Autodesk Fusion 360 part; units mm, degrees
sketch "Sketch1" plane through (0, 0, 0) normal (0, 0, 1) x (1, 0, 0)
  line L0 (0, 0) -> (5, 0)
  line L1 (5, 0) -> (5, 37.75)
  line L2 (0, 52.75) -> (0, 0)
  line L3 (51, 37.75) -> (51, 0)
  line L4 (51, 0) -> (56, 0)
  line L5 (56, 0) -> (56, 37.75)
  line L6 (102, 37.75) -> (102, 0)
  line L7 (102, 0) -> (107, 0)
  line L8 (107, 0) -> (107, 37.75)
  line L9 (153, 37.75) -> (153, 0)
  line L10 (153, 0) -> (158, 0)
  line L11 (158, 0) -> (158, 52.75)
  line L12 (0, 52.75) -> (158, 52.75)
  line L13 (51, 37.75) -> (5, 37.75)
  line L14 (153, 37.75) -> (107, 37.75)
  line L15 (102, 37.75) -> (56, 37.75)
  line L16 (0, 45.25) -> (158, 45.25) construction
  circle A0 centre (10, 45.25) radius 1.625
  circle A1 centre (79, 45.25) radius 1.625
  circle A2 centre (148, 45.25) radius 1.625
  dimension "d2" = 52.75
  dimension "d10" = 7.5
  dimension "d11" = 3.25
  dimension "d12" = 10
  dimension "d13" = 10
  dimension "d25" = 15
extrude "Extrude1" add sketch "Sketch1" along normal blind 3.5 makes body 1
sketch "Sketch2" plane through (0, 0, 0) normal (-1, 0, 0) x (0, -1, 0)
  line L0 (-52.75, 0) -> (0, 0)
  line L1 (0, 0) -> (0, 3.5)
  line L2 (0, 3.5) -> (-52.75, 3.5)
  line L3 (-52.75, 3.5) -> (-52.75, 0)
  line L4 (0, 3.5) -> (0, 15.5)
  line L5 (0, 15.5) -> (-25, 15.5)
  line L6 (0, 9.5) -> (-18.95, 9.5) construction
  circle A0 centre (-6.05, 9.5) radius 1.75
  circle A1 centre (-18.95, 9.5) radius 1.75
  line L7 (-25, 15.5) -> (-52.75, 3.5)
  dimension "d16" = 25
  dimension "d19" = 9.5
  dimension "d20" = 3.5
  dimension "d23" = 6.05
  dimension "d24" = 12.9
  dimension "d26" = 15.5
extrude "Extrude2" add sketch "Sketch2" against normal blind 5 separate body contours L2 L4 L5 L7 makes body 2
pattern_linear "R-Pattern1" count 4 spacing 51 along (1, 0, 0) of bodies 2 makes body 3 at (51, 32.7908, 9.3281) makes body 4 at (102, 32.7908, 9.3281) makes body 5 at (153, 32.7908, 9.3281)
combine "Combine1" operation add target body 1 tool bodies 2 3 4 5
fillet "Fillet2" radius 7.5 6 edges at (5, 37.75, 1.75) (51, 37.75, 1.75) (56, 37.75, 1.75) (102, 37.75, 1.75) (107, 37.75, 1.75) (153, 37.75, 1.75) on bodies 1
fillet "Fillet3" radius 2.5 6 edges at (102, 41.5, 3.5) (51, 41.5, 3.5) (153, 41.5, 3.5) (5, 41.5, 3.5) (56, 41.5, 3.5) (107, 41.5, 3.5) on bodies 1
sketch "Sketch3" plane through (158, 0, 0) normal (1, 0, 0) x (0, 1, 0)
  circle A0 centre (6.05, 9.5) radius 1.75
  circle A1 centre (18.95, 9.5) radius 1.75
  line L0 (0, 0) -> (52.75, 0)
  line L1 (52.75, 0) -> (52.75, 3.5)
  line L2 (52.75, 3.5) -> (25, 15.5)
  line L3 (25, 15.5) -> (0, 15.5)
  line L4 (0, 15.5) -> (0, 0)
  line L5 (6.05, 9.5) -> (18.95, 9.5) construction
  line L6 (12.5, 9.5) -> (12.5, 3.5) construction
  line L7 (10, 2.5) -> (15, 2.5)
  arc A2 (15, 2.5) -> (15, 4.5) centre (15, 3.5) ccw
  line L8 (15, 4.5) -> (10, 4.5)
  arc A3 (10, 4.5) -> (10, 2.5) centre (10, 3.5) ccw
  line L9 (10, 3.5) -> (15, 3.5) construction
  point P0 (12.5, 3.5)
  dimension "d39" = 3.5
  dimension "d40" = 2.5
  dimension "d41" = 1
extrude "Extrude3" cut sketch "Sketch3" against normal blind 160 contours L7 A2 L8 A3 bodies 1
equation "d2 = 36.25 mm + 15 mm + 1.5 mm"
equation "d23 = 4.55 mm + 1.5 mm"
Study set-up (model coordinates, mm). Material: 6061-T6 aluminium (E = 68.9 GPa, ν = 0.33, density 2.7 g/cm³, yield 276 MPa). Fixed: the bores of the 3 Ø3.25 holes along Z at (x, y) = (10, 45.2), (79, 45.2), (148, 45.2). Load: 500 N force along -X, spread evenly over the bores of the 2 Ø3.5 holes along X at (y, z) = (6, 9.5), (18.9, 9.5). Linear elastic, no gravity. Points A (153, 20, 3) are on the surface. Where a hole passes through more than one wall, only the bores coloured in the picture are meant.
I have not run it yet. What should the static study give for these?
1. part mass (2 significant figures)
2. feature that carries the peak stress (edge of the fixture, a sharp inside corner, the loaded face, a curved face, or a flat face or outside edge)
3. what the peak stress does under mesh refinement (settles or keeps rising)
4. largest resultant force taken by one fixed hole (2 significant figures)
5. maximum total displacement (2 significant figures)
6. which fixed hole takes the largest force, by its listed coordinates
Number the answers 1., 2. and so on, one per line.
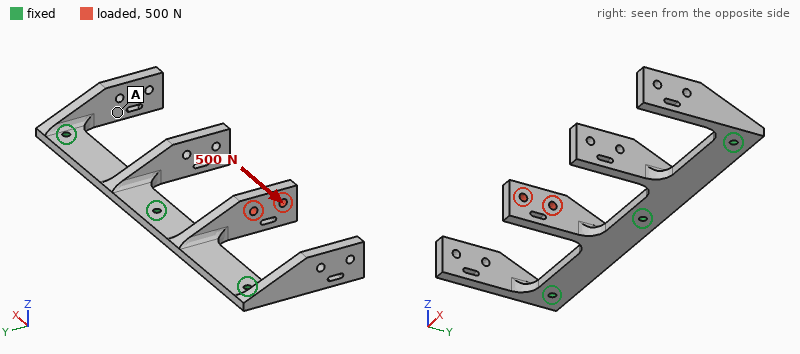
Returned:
1. 54 g
2. a sharp inside corner
3. keeps rising
4. 400 N
5. 0.70 mm
6. (79, 45.2)
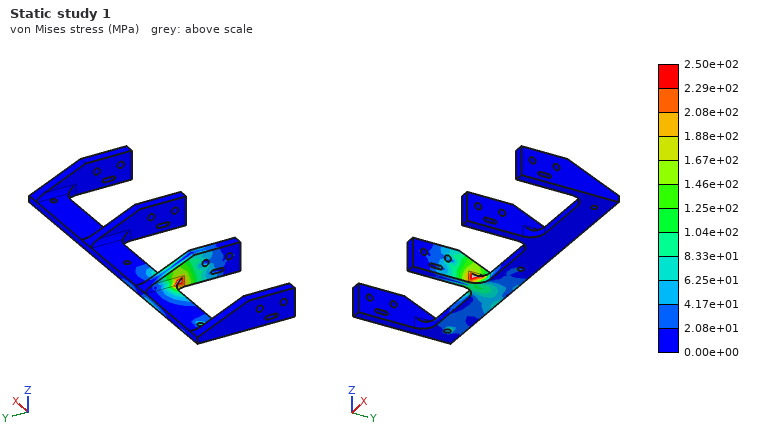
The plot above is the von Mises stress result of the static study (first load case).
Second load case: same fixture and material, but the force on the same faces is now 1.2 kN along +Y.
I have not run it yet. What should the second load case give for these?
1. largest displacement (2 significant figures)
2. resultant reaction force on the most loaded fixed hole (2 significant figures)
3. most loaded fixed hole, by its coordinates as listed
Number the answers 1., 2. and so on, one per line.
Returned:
1. 1.3 mm
2. 900 N
3. (79, 45.2)
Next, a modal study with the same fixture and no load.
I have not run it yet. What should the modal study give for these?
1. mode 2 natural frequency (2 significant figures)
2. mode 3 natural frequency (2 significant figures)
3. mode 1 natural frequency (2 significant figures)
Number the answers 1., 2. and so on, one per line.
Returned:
1. 1100 Hz
2. 1700 Hz
3. 1100 Hz
